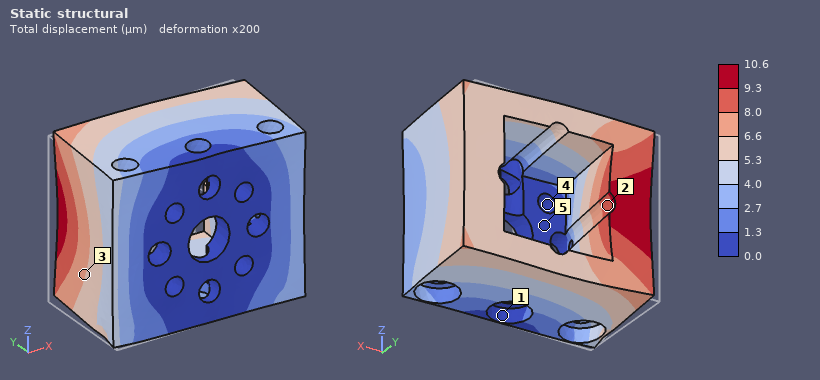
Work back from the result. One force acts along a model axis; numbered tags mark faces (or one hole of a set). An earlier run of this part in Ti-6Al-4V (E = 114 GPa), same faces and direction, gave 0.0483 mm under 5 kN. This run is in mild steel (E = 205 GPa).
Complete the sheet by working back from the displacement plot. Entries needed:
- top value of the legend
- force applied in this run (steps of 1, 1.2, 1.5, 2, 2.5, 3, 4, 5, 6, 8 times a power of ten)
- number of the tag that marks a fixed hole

10.6 µm
2 kN
4
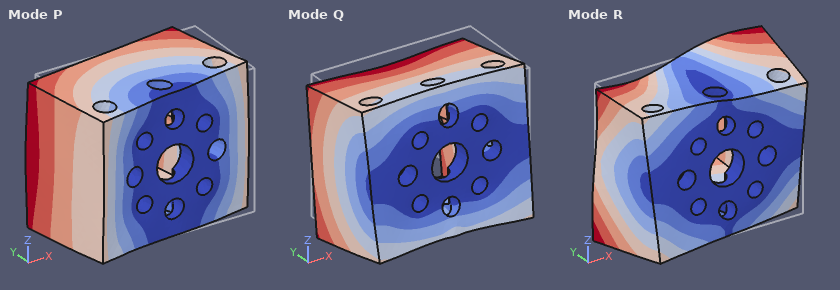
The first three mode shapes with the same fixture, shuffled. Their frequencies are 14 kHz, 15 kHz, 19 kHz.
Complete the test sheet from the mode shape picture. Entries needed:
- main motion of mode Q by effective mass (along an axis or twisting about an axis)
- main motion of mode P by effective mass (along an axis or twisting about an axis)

along Z
along X
